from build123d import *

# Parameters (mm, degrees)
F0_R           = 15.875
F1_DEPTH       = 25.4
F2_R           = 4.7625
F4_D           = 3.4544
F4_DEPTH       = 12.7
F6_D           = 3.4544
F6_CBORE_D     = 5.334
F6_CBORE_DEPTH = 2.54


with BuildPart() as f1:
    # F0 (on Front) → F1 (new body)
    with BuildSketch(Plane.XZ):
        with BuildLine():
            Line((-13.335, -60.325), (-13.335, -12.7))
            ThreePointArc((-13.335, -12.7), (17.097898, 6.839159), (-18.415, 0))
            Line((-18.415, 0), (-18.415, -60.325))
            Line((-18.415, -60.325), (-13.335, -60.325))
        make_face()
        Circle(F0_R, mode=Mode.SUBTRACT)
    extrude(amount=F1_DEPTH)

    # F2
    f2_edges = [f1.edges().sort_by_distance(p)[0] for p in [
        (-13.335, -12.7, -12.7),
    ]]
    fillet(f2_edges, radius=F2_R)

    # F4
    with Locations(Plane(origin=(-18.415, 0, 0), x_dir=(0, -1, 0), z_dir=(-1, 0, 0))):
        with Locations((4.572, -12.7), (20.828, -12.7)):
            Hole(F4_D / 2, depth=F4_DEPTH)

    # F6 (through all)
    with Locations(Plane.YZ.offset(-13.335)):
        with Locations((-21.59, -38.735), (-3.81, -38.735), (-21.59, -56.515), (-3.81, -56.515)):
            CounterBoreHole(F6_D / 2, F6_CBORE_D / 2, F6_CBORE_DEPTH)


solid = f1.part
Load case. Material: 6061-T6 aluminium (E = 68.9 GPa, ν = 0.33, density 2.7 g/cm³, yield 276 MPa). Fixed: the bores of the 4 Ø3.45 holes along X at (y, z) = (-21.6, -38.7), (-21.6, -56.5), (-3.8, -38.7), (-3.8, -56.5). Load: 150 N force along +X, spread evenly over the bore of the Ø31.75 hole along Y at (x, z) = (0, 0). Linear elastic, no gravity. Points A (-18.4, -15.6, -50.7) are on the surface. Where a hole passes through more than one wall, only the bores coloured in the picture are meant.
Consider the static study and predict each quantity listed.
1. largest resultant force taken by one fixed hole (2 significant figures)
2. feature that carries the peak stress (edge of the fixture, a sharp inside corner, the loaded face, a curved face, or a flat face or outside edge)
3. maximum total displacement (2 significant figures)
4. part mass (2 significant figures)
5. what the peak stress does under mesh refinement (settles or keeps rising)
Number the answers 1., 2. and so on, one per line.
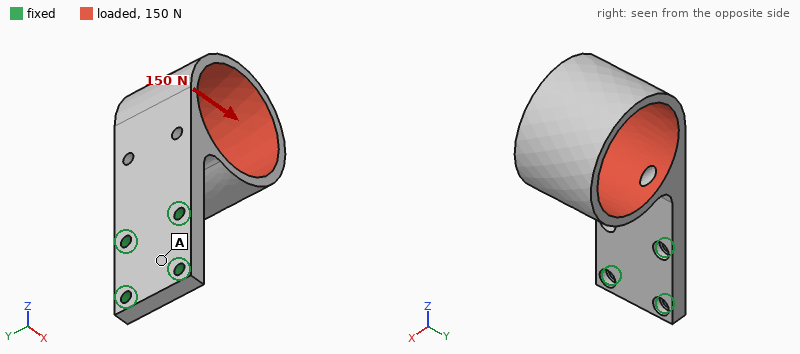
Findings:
1. 280 N
2. edge of the fixture
3. 0.36 mm
4. 36 g
5. keeps rising
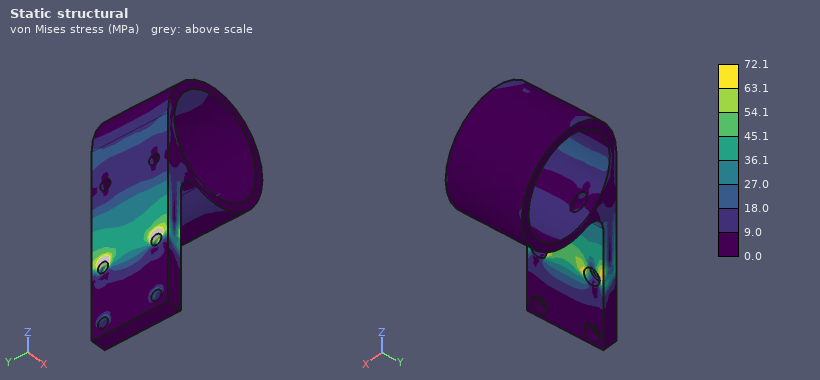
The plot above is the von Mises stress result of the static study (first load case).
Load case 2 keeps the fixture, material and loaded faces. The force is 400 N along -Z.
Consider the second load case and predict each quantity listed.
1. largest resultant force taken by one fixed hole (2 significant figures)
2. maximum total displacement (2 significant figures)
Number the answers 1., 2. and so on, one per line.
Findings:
1. 290 N
2. 0.60 mm
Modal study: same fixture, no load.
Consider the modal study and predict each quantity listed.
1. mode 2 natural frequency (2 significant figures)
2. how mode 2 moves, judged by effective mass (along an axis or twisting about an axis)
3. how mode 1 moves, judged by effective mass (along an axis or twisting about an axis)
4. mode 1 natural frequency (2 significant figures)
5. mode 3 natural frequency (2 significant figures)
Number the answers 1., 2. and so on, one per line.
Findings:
1. 1900 Hz
2. along Y
3. along X
4. 750 Hz
5. 3000 Hz
